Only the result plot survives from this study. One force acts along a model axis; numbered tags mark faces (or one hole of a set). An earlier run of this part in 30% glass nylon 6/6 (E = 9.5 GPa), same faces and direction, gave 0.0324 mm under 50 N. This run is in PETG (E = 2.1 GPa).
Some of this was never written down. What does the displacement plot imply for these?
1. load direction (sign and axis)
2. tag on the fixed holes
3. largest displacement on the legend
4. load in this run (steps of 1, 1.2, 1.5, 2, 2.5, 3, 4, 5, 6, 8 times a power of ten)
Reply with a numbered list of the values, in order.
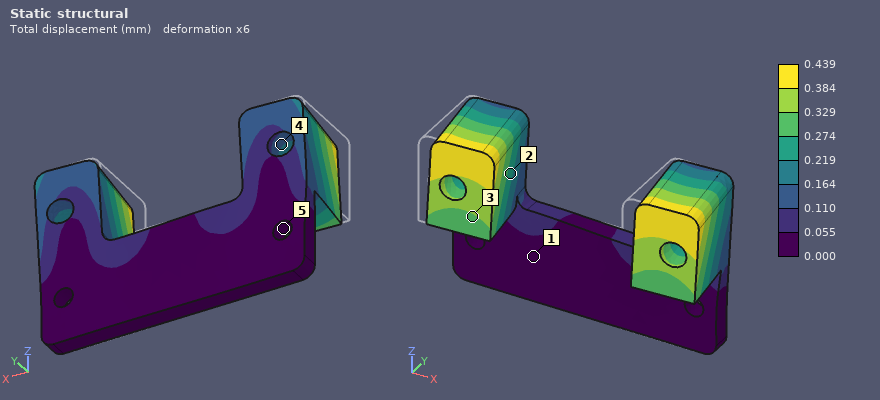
1. +X
2. 5
3. 0.439 mm
4. 150 N
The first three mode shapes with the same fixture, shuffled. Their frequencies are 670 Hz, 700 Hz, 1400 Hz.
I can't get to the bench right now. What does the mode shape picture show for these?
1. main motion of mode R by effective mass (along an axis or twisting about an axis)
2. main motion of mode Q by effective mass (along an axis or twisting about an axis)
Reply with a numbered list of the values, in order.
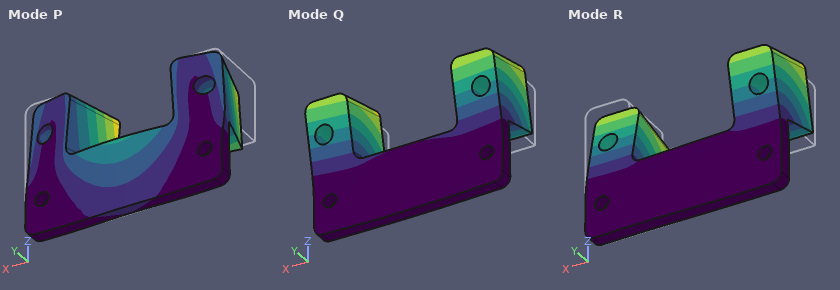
1. twisting about Z
2. along Y
